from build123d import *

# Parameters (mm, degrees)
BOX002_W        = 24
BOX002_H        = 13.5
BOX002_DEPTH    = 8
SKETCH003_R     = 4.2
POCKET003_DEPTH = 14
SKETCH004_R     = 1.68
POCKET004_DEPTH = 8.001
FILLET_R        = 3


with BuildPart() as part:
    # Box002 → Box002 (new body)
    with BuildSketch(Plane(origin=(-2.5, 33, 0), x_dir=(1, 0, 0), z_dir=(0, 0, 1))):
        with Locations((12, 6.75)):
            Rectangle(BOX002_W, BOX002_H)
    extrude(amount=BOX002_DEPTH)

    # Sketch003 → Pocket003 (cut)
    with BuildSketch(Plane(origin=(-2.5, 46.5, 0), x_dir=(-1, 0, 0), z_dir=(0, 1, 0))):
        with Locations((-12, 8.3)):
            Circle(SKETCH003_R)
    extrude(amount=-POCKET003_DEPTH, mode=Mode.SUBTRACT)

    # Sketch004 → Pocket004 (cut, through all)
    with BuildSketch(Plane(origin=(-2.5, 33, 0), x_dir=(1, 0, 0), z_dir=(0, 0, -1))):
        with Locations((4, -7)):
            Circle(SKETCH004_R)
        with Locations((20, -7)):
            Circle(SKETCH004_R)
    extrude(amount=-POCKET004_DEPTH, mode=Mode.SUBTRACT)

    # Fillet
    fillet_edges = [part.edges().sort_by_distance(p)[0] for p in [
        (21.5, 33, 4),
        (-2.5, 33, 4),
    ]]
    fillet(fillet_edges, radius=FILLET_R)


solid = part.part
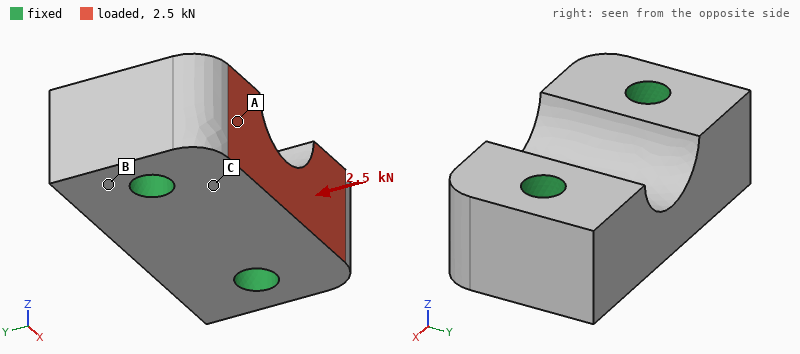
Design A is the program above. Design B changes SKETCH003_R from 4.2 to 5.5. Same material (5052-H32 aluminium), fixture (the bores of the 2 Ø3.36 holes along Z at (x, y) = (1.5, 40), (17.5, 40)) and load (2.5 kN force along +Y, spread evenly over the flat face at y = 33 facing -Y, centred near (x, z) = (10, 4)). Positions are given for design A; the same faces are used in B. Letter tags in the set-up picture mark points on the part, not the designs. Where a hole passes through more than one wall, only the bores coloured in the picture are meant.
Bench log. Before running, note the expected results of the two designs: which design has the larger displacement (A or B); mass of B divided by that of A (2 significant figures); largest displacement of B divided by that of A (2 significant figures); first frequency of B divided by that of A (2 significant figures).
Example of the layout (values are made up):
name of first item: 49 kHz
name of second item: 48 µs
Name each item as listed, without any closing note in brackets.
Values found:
which design has the larger displacement: B
mass of B divided by that of A: 0.88
largest displacement of B divided by that of A: 1.2
first frequency of B divided by that of A: 1.0
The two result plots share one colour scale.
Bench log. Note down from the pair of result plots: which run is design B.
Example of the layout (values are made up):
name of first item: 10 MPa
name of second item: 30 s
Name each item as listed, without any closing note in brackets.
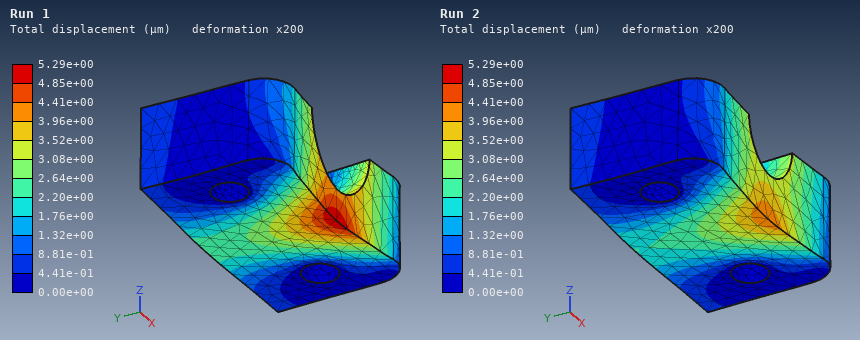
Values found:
which run is design B: Run 1
